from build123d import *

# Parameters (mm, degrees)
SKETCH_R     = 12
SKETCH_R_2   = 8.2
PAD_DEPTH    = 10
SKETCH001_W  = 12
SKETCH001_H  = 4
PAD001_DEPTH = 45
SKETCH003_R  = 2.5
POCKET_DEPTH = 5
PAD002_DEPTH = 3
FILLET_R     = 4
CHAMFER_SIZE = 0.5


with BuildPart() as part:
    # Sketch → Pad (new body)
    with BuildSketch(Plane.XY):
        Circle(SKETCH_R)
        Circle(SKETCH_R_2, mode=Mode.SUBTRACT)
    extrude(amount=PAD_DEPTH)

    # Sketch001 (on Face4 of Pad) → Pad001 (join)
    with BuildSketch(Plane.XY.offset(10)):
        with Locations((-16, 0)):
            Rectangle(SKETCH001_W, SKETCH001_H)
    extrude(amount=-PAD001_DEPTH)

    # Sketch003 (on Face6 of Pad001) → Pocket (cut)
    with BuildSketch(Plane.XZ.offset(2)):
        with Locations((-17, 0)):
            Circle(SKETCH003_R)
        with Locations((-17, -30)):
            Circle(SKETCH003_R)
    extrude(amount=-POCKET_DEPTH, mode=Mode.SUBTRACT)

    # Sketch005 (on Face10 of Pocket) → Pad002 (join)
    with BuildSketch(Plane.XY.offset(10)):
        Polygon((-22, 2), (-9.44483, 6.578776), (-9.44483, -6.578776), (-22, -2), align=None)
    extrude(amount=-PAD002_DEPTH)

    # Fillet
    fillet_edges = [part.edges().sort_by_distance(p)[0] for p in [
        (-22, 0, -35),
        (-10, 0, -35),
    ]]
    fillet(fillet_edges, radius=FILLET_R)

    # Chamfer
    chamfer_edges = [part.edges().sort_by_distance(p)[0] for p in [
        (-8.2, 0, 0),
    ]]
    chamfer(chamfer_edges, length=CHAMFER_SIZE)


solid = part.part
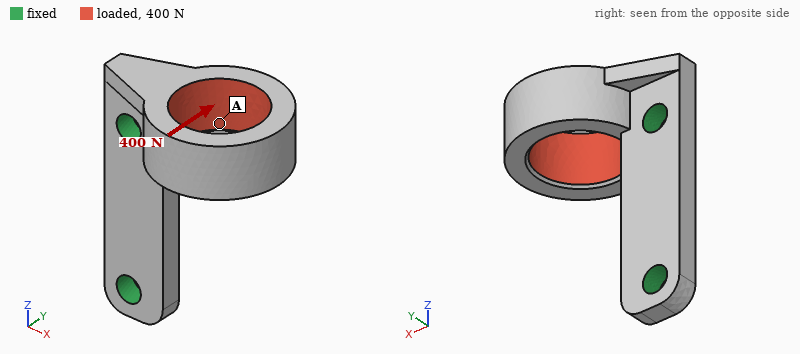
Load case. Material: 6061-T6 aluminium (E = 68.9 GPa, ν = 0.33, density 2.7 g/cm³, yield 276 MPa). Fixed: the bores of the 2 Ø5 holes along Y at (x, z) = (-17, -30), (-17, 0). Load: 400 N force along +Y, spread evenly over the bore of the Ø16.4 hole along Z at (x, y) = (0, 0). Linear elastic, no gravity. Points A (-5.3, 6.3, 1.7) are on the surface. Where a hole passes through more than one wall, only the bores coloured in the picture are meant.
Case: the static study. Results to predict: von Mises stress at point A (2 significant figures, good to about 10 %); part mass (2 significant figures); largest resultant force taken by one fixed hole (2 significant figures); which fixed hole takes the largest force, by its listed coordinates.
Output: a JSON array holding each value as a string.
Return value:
["32 MPa", "12 g", "420 N", "(-17, 0)"]
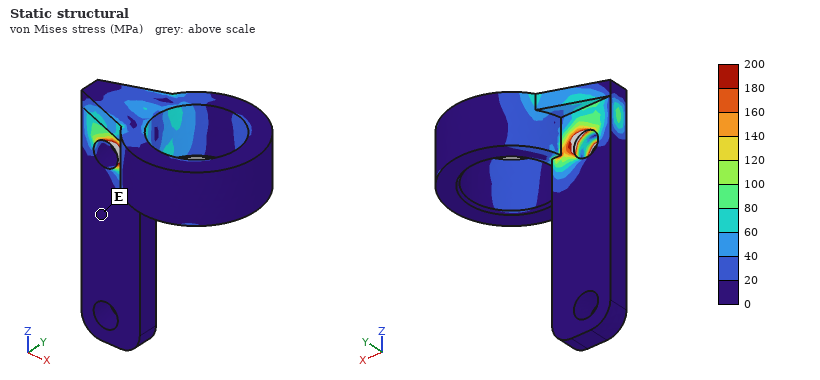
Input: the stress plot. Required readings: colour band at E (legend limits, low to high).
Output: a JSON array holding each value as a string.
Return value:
["0 to 20 MPa"]
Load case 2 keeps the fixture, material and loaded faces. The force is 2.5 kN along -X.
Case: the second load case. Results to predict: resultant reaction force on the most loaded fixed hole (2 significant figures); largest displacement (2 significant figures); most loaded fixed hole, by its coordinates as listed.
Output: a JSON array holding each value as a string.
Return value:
["2.6 kN", "80 µm", "(-17, 0)"]
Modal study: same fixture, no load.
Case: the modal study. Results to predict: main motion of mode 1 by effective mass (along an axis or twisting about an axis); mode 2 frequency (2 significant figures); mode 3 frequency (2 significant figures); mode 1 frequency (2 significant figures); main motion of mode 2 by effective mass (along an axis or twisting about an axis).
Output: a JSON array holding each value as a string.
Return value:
["along Y", "5300 Hz", "8800 Hz", "3100 Hz", "along Z"]
